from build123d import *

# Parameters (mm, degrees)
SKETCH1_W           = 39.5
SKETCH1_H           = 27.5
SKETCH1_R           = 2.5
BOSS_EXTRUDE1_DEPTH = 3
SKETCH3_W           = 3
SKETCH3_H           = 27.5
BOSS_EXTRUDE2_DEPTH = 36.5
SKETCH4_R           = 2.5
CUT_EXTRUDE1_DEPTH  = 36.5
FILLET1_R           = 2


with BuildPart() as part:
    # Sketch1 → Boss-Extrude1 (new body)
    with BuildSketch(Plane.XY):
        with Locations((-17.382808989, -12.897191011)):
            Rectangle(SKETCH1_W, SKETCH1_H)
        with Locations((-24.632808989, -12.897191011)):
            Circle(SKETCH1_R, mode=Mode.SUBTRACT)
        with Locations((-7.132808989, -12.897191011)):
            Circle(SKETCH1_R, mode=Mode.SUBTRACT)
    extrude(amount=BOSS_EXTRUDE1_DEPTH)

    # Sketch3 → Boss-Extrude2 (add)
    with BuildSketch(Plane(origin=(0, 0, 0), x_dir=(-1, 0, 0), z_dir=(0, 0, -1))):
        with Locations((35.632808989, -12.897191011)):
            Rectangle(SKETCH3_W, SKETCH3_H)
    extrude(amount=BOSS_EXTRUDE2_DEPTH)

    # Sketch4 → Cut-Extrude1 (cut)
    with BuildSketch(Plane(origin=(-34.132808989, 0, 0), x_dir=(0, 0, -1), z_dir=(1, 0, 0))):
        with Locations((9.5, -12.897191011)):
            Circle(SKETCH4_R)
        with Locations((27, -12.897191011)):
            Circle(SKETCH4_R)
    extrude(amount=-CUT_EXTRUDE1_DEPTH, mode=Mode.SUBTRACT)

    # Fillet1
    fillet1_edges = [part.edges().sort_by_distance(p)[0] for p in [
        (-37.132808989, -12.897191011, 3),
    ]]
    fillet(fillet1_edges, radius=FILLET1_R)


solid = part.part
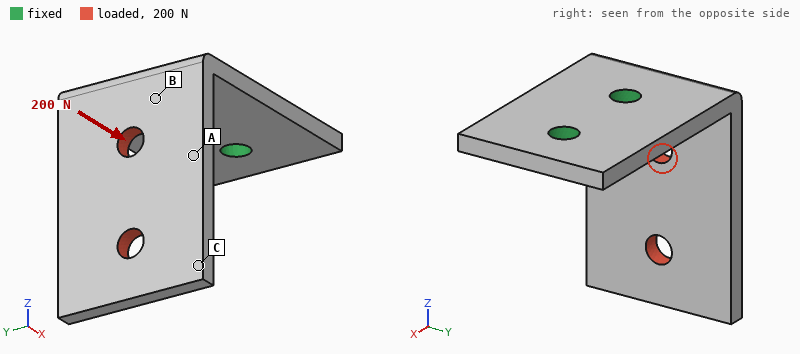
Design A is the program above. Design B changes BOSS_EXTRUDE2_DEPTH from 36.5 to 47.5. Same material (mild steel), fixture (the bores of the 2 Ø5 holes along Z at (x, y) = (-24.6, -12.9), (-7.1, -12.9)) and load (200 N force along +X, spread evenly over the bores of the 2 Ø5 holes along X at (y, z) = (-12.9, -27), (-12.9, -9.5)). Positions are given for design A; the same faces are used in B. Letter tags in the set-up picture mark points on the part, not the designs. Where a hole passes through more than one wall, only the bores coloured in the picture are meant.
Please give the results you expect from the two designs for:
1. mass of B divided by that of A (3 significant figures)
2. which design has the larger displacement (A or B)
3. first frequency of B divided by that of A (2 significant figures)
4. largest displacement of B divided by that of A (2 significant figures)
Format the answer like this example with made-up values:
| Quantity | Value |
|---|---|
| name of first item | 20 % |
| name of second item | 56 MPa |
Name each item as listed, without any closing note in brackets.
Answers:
| Quantity | Value |
|---|---|
| mass of B divided by that of A | 1.15 |
| which design has the larger displacement | B |
| first frequency of B divided by that of A | 0.63 |
| largest displacement of B divided by that of A | 1.3 |
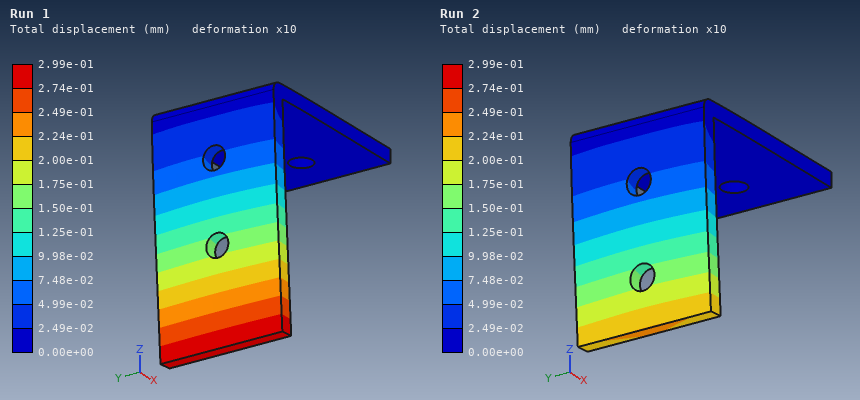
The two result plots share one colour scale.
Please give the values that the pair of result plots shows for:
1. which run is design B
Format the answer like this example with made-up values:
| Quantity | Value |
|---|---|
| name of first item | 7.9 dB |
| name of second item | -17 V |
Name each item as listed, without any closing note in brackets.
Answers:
| Quantity | Value |
|---|---|
| which run is design B | Run 1 |
